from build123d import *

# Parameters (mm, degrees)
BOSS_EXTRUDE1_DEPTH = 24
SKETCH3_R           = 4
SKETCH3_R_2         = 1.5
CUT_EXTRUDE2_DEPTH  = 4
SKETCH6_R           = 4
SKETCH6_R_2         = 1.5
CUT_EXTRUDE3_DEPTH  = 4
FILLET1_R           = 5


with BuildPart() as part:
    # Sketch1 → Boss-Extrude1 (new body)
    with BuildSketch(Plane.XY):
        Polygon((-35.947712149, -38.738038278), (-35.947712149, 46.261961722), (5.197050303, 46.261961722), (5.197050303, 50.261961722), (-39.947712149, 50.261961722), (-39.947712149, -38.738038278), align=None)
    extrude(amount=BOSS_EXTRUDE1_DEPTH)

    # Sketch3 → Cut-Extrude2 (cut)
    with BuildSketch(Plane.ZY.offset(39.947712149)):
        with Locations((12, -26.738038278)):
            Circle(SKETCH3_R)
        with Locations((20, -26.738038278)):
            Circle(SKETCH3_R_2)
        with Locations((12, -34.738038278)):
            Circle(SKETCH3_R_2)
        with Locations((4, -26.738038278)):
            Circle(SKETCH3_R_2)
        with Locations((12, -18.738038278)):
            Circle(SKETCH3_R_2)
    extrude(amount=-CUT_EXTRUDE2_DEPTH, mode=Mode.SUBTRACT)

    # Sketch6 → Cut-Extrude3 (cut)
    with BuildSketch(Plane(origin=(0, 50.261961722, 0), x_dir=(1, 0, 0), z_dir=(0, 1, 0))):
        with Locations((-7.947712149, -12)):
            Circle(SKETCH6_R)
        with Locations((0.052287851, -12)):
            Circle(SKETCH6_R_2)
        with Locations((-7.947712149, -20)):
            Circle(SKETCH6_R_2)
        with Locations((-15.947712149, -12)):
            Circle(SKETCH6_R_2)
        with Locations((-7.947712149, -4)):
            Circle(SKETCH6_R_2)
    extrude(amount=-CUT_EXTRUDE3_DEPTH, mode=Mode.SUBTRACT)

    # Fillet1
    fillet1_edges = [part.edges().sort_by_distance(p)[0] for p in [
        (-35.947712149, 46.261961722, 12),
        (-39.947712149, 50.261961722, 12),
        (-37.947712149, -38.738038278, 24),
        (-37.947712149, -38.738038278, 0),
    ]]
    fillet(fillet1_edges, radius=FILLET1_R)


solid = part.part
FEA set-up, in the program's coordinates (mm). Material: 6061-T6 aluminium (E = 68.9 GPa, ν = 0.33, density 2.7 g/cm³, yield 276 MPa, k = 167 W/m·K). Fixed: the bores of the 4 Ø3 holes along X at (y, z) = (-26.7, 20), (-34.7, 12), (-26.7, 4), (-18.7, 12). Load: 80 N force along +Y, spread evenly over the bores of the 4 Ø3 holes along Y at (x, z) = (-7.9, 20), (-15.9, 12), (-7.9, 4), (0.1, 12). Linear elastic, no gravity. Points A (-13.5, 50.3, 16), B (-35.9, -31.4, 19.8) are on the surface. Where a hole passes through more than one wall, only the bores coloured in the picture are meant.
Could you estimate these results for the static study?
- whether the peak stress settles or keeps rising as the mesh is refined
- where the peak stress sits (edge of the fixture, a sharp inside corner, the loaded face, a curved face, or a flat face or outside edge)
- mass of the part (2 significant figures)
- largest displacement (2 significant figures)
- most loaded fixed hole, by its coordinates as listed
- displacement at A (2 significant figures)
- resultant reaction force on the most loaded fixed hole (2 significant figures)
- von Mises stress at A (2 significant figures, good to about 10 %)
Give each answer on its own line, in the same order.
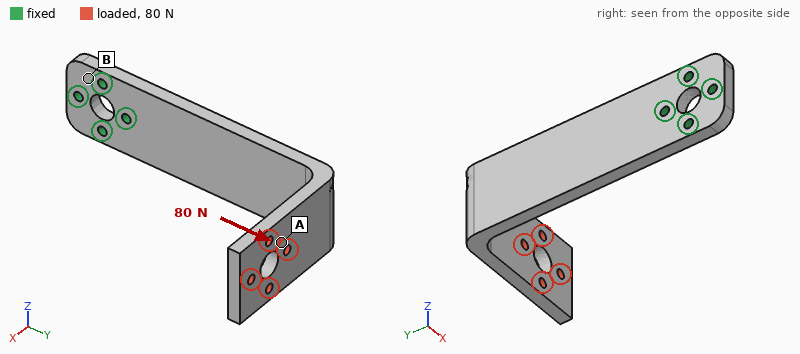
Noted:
keeps rising
edge of the fixture
32 g
1.1 mm
(-18.7, 12)
0.80 mm
170 N
8.9 MPa
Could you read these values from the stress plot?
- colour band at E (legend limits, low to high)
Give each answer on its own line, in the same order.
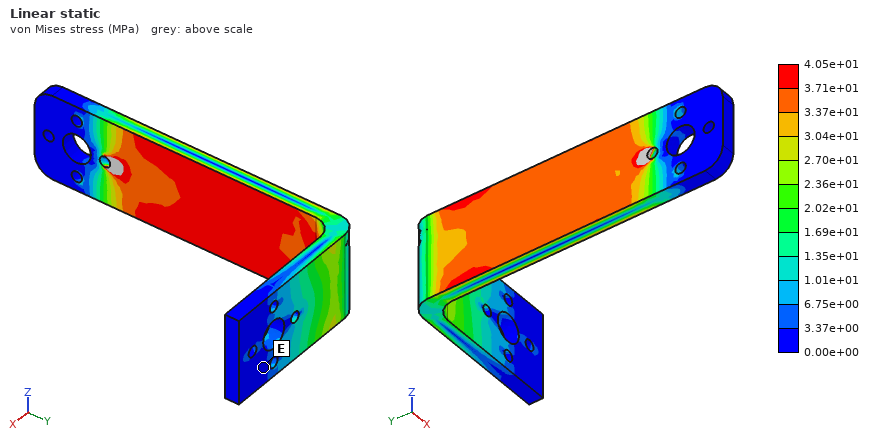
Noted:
0.00e+00 to 3.37e+00 MPa
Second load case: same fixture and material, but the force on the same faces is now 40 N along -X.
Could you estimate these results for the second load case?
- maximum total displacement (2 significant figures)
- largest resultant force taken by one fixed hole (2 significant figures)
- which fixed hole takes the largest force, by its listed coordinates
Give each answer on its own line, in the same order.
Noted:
0.65 mm
200 N
(-18.7, 12)
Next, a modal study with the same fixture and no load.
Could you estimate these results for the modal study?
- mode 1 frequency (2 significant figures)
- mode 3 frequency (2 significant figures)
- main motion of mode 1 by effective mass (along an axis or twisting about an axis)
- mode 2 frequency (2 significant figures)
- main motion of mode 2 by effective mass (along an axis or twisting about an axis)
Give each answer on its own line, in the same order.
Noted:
350 Hz
1300 Hz
along X
800 Hz
along Z
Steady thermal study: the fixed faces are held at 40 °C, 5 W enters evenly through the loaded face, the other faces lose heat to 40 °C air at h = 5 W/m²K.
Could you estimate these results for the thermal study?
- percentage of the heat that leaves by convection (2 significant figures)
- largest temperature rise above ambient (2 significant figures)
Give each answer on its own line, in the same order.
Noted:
9.7 %
29 K
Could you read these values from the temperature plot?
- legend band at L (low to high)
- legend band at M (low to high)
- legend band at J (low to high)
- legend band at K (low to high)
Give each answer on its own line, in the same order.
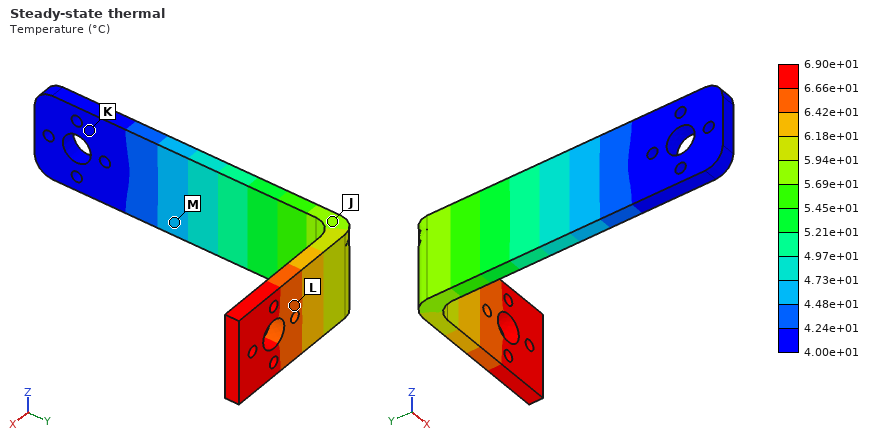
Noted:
6.42e+01 to 6.66e+01 °C
4.48e+01 to 4.73e+01 °C
5.69e+01 to 5.94e+01 °C
4.00e+01 to 4.24e+01 °C
